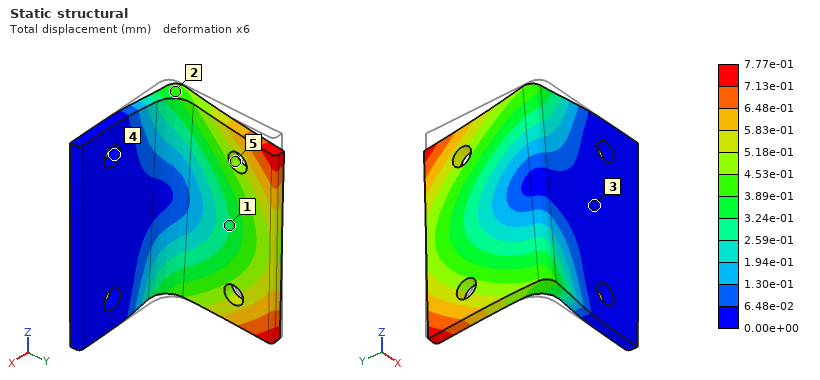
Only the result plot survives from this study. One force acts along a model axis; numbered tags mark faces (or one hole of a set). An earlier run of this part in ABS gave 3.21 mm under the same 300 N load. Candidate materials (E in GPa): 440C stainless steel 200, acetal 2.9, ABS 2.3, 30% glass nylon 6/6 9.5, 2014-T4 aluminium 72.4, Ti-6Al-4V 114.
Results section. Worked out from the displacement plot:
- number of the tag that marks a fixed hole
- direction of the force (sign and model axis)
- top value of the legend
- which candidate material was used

4
-Z
7.77e-01 mm
30% glass nylon 6/6
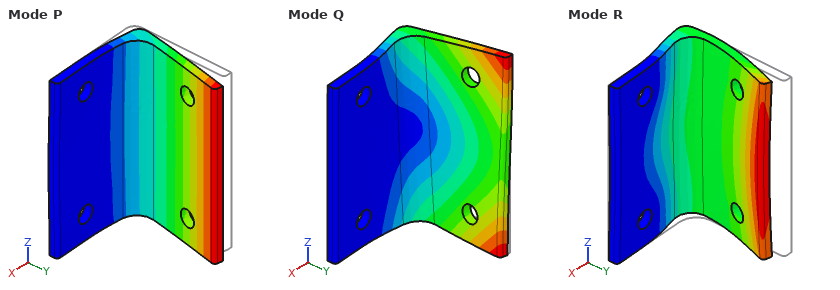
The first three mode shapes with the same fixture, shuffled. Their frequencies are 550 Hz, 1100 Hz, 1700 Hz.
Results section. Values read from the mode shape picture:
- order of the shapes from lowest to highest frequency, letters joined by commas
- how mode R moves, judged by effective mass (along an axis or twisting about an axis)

P, Q, R
along Y
